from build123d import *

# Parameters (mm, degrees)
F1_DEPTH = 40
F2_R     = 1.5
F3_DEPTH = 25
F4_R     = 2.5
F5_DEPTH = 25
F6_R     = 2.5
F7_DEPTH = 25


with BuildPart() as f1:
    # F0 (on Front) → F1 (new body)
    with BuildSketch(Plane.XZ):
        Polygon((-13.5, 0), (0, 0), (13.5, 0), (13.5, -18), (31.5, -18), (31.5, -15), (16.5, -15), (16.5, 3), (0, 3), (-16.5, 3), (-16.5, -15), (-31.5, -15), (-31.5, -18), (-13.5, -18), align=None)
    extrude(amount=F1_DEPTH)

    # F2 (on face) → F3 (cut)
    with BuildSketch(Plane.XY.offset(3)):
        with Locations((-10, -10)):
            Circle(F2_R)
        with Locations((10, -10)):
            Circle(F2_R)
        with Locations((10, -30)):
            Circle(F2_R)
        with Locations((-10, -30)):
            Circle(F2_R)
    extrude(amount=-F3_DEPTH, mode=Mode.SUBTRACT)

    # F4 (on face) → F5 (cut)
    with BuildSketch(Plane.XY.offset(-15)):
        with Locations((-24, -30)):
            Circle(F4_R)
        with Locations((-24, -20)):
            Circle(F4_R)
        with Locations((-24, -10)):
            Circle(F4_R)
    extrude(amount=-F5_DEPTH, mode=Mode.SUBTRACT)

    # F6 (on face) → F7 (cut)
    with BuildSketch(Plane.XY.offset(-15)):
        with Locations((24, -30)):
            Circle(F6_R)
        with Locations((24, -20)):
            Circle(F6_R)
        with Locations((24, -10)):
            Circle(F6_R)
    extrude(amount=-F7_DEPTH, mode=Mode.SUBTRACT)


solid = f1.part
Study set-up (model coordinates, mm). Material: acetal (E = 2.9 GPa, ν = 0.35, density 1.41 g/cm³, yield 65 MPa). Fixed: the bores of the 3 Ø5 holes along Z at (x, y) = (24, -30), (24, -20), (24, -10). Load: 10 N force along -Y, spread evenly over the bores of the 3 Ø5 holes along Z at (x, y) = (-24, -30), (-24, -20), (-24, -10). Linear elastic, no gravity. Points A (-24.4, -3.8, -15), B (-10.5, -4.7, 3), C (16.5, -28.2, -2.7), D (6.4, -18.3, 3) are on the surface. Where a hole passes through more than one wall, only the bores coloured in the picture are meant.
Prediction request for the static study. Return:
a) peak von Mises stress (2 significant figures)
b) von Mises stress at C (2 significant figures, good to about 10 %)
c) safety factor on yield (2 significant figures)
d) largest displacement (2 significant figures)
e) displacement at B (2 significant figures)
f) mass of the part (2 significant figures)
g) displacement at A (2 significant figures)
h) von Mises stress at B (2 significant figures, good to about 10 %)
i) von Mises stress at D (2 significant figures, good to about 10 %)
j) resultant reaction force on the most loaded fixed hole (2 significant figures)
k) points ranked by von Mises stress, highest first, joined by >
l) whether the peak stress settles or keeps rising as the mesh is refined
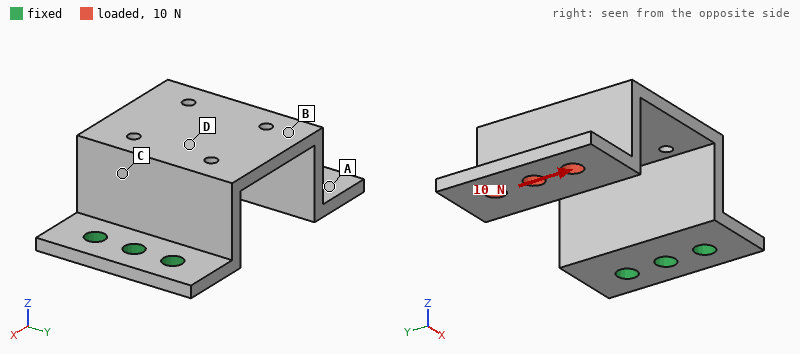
5.4 MPa
3.7 MPa
12
0.86 mm
0.36 mm
16 g
0.72 mm
2.1 MPa
2.8 MPa
19 N
C > D > B > A
settles
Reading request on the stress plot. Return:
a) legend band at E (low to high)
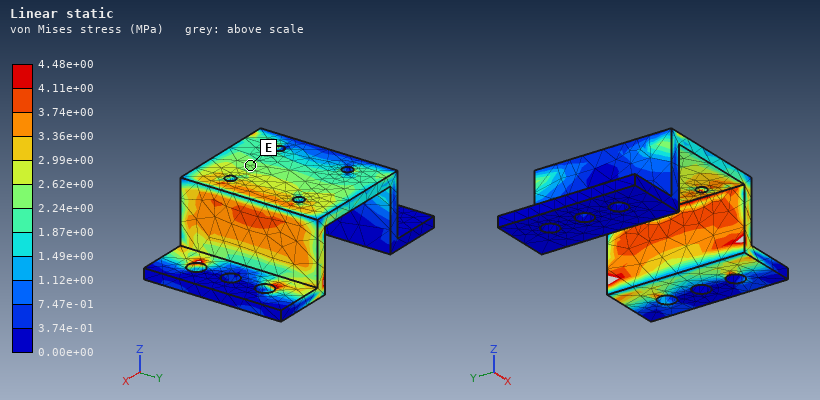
2.24e+00 to 2.62e+00 MPa
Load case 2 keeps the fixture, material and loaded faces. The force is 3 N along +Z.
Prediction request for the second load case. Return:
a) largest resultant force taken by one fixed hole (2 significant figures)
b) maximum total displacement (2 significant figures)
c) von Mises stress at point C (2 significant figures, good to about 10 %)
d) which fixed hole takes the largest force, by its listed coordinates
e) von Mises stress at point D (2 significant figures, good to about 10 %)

1.9 N
0.82 mm
1.6 MPa
(24, -20)
1.4 MPa
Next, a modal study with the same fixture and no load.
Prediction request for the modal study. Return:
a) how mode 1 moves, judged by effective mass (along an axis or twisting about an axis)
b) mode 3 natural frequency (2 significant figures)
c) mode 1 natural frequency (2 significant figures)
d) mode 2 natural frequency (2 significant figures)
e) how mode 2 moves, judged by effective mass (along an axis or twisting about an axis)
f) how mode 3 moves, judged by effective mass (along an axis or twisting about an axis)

along Z
420 Hz
150 Hz
270 Hz
along Y
along X
